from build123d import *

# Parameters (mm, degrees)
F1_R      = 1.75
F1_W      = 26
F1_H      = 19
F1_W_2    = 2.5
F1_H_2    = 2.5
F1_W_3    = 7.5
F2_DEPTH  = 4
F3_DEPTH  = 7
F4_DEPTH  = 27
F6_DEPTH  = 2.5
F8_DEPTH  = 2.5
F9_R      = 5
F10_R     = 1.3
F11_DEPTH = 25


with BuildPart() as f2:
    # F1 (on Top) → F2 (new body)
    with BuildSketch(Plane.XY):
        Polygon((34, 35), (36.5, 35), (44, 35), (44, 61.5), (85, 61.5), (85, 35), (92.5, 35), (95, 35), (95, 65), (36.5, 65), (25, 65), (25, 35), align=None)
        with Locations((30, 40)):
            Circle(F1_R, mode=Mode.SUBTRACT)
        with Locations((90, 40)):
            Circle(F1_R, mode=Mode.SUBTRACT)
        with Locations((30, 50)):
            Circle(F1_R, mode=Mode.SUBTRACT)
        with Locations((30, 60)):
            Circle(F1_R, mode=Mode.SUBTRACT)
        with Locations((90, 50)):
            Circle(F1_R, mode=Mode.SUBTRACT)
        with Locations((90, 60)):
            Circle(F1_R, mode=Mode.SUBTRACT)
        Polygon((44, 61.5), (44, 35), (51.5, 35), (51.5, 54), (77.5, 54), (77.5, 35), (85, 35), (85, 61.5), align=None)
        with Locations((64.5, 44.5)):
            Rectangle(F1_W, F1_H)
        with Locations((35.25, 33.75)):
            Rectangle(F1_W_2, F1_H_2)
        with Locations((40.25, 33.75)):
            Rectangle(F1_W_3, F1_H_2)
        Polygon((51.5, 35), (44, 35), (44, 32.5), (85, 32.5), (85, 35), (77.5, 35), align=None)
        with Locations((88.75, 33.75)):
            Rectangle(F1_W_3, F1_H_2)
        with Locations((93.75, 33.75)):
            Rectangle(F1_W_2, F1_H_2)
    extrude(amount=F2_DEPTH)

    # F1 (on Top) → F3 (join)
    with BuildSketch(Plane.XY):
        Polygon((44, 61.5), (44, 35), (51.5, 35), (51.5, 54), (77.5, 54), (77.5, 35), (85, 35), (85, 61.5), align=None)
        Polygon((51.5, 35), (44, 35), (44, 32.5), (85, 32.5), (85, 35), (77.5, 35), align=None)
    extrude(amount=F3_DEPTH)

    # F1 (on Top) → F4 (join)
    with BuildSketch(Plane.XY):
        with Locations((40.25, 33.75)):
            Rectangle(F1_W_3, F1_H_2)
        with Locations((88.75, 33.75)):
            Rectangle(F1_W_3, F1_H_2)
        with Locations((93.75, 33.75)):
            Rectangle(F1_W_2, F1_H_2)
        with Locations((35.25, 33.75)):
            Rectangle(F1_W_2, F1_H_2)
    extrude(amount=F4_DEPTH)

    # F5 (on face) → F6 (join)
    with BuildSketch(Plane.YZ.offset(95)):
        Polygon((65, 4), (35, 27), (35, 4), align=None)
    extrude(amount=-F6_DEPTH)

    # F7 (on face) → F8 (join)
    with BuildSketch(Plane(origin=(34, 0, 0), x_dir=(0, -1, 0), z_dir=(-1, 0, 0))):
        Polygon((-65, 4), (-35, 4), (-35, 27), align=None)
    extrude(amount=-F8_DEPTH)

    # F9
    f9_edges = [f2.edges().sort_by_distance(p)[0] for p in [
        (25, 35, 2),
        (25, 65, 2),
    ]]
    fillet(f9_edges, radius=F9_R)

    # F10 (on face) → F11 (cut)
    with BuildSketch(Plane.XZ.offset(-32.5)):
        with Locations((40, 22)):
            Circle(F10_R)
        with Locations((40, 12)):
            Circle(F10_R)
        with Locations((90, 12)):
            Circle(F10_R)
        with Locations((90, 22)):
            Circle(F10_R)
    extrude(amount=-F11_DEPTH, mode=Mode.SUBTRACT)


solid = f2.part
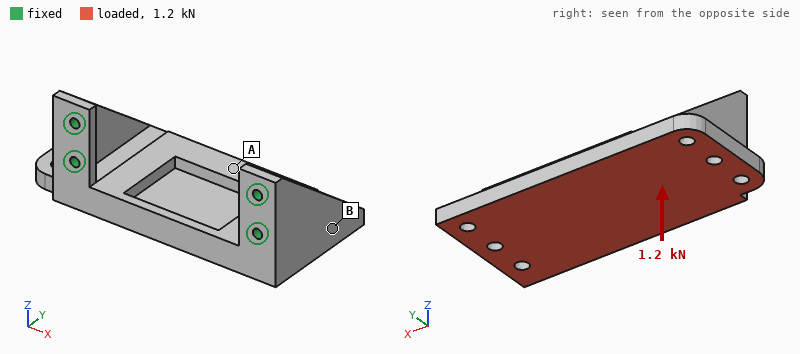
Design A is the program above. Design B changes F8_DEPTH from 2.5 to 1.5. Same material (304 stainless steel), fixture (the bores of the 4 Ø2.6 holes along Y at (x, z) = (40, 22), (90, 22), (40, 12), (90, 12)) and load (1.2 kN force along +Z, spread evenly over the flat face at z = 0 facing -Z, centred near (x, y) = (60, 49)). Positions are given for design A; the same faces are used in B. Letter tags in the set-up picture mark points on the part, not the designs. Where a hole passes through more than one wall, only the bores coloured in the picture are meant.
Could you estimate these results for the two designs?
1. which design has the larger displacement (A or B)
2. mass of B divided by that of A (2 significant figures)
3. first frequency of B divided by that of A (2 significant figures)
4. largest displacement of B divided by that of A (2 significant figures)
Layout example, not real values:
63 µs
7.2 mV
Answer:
B
0.97
0.92
1.2
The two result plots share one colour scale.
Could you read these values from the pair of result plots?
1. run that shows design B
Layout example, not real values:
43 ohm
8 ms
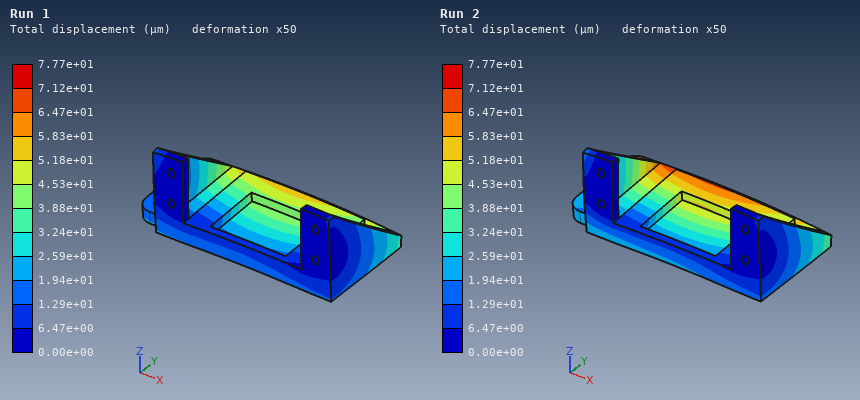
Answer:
Run 2
